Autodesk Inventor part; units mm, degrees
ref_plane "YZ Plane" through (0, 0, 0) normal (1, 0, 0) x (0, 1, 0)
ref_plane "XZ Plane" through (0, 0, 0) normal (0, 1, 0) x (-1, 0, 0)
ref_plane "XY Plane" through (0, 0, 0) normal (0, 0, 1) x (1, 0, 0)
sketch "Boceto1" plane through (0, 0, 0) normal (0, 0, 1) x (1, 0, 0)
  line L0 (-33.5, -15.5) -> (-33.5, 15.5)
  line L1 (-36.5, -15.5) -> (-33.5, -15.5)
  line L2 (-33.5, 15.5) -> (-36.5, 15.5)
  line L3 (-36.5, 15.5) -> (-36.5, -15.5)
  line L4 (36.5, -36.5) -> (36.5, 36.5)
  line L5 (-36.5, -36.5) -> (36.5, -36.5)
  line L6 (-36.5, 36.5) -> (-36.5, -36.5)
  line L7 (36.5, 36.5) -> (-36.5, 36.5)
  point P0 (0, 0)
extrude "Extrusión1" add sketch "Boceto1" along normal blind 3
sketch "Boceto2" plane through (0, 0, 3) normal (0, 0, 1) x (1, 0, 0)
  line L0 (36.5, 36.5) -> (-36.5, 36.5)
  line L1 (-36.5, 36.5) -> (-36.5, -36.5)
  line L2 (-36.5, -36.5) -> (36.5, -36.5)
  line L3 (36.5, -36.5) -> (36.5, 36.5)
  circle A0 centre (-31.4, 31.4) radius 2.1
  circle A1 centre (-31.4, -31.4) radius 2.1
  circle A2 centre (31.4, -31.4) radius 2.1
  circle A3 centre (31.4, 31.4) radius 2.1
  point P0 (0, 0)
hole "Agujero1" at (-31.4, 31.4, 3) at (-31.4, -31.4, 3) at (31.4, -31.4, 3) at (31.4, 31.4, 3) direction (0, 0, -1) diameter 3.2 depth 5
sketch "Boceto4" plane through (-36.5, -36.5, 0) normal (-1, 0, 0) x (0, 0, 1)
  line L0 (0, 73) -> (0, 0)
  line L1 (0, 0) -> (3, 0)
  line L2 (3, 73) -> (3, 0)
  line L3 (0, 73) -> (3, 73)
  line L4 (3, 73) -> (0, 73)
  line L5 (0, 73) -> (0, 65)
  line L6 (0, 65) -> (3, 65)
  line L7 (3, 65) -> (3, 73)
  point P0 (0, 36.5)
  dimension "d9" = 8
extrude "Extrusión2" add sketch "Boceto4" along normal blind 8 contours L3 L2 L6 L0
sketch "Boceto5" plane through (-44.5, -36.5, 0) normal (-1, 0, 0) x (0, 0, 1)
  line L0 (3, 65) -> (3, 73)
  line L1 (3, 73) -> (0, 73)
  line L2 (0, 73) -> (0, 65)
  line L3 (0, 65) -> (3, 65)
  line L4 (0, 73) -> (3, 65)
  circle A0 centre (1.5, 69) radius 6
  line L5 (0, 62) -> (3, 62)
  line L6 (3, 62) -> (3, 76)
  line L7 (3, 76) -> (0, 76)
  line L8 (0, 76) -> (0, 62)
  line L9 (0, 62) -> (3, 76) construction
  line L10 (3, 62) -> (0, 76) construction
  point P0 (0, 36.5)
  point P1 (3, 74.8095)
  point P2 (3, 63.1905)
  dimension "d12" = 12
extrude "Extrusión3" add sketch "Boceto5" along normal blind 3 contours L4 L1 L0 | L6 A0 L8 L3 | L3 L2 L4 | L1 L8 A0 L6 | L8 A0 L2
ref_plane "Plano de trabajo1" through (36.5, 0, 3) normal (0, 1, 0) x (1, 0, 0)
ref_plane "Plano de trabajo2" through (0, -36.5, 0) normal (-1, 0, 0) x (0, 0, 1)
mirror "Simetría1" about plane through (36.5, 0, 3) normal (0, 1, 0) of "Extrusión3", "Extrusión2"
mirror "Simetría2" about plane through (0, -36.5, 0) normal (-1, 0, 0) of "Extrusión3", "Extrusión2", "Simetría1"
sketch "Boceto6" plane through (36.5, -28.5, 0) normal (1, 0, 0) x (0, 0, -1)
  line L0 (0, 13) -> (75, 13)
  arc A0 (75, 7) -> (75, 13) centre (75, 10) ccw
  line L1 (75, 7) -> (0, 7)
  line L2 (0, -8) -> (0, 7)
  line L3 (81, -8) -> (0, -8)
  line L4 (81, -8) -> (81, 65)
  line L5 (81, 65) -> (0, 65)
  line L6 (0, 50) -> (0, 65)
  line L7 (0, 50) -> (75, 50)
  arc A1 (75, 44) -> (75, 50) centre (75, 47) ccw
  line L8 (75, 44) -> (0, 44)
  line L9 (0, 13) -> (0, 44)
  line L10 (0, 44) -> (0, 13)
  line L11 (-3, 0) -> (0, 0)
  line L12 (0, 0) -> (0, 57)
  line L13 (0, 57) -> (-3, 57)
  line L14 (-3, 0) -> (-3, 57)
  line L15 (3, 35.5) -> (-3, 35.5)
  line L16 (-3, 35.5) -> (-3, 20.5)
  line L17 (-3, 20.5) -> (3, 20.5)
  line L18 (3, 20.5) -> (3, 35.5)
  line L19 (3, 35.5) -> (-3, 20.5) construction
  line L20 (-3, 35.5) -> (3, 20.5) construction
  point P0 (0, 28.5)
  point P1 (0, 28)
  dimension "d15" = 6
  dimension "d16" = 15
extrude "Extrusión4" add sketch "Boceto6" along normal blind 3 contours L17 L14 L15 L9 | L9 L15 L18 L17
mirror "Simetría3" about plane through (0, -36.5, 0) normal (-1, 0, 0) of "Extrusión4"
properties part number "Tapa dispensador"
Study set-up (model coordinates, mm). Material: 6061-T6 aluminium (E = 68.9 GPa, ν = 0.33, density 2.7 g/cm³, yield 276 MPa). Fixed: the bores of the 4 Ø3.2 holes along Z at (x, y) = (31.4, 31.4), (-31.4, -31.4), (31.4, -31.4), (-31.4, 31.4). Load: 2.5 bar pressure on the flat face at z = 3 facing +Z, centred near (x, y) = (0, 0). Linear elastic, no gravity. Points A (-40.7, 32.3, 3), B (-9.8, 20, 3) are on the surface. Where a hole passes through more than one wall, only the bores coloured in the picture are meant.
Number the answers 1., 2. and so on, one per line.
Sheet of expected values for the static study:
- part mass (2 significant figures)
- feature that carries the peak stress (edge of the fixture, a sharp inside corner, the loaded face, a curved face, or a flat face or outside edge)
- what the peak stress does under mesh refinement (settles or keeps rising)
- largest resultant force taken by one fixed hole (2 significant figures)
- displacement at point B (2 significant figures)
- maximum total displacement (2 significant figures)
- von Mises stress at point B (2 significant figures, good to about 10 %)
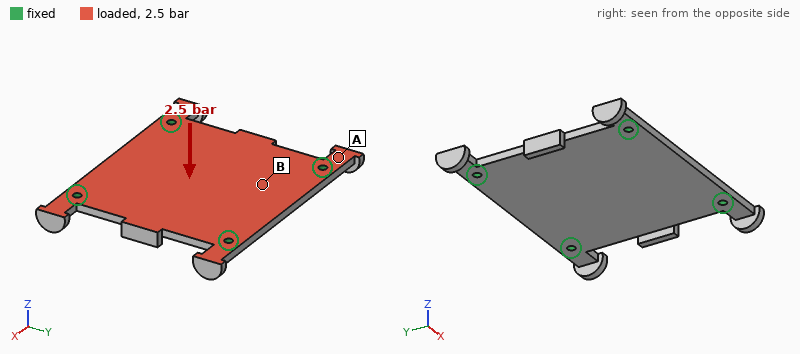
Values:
1. 49 g
2. edge of the fixture
3. keeps rising
4. 360 N
5. 0.12 mm
6. 0.18 mm
7. 27 MPa
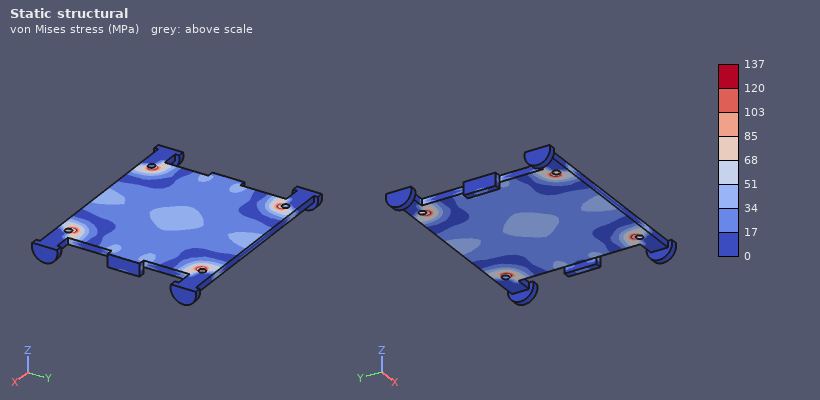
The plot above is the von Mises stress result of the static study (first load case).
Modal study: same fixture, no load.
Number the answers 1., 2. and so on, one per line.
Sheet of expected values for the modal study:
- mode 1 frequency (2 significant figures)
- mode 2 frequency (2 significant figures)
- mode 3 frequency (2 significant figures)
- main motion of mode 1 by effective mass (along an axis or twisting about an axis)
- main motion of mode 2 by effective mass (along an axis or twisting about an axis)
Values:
1. 2500 Hz
2. 4000 Hz
3. 4300 Hz
4. along Z
5. twisting about Y
